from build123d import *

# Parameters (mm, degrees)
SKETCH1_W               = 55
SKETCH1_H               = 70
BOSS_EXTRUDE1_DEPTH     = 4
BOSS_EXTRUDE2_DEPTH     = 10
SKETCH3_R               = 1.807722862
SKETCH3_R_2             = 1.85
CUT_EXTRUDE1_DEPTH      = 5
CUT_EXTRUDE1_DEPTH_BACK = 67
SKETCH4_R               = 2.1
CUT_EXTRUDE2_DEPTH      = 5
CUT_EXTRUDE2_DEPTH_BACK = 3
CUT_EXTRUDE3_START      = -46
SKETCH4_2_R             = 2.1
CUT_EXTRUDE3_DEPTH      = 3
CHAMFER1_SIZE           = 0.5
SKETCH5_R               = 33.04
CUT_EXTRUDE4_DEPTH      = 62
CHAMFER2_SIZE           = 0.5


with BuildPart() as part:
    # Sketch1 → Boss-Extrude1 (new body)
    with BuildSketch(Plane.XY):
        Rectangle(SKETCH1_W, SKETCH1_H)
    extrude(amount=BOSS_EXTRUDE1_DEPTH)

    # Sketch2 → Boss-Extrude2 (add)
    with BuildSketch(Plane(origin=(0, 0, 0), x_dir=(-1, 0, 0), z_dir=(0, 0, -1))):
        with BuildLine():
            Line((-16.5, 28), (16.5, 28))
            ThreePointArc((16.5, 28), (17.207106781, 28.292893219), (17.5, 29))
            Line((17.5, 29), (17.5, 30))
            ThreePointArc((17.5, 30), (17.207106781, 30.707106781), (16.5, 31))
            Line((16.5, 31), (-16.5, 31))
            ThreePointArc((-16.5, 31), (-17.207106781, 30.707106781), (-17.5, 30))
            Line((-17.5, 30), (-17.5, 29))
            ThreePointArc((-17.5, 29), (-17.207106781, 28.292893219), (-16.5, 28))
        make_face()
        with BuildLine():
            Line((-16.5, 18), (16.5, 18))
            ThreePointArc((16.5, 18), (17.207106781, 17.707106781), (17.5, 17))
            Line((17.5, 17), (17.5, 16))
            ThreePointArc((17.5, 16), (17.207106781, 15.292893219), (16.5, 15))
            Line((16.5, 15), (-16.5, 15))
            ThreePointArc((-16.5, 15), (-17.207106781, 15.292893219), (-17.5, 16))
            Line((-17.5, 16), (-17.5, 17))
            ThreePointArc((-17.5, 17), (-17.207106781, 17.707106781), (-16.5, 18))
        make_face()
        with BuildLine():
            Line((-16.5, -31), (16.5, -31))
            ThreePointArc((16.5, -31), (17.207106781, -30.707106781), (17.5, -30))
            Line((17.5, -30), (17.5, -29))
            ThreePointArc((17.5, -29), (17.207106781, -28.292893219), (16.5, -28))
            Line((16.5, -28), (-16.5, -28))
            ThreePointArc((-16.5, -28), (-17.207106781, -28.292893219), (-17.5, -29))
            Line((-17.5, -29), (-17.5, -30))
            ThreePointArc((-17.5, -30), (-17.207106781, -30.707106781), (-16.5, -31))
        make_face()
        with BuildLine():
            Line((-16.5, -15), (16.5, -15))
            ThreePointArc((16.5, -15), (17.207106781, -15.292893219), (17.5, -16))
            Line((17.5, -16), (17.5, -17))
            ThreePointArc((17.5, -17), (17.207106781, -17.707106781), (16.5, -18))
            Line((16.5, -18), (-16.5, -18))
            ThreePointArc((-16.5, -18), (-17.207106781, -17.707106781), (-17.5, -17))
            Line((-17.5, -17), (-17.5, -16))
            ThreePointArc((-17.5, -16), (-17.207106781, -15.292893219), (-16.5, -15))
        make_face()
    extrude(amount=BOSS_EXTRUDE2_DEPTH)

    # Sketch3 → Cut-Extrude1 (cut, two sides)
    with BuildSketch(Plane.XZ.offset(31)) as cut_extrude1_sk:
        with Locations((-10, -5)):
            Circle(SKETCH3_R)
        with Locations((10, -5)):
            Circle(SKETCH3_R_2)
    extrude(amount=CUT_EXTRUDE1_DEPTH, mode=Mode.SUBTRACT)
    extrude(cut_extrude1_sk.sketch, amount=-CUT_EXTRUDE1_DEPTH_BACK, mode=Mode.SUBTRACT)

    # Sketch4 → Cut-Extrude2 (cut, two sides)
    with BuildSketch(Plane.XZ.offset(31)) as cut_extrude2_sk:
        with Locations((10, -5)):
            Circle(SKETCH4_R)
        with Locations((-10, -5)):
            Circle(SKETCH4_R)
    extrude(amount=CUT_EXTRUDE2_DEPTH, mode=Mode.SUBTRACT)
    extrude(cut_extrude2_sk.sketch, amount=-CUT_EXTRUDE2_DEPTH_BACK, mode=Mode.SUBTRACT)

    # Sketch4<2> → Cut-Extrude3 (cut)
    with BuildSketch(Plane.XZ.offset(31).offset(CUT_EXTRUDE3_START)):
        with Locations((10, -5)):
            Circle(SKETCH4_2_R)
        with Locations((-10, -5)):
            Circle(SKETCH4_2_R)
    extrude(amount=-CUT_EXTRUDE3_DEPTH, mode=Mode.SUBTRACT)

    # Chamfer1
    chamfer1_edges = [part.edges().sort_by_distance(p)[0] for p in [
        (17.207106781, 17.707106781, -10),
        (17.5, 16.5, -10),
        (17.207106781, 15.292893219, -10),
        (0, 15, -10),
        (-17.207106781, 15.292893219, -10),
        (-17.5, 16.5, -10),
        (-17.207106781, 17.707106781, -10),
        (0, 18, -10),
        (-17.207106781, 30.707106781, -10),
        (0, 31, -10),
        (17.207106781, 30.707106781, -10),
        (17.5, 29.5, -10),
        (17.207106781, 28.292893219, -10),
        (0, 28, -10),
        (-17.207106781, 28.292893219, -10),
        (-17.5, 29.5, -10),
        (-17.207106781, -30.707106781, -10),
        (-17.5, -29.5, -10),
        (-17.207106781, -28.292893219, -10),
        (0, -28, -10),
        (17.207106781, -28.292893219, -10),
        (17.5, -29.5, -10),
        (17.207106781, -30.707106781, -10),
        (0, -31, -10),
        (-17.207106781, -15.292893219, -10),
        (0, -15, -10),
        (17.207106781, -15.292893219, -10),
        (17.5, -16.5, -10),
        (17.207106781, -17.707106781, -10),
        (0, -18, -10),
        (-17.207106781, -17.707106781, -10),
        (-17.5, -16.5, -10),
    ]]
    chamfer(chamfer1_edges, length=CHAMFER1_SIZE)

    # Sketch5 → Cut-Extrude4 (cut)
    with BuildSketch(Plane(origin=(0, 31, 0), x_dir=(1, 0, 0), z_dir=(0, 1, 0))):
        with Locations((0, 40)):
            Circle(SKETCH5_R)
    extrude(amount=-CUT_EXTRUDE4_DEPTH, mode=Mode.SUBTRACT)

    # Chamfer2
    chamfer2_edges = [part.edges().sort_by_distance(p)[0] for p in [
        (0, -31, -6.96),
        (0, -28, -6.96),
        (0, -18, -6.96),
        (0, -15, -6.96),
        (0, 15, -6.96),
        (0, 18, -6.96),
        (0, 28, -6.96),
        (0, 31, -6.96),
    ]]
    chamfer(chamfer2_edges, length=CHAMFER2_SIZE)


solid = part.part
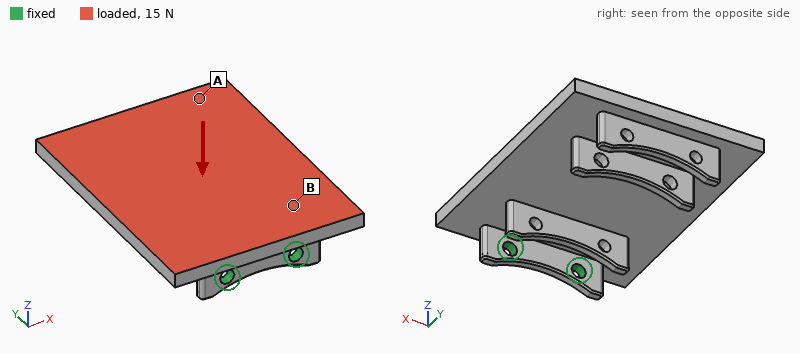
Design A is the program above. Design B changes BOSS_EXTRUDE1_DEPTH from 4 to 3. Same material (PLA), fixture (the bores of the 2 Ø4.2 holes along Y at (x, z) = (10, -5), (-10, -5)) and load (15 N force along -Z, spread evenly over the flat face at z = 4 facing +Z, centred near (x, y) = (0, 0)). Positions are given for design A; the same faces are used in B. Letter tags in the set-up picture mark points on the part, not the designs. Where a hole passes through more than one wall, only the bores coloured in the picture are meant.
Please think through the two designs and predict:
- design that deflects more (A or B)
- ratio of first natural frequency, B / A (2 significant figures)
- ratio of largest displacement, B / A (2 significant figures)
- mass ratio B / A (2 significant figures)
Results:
B
0.89
1.6
0.79
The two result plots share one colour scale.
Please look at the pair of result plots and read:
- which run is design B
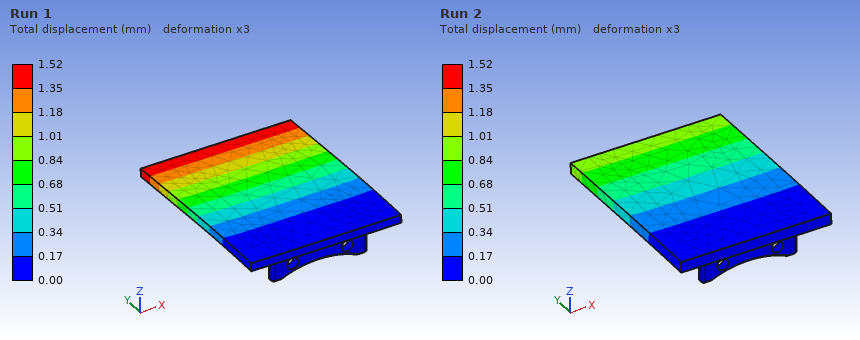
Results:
Run 1
